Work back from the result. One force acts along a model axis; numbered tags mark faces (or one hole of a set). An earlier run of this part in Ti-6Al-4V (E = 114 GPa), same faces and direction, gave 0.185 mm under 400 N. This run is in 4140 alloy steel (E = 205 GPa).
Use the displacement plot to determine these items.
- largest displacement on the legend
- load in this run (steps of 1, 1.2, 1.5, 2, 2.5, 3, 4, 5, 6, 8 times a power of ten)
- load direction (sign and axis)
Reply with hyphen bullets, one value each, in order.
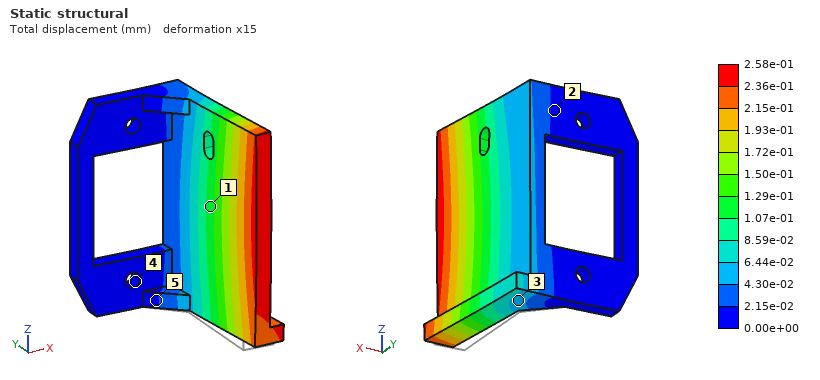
- 2.58e-01 mm
- 1 kN
- +X
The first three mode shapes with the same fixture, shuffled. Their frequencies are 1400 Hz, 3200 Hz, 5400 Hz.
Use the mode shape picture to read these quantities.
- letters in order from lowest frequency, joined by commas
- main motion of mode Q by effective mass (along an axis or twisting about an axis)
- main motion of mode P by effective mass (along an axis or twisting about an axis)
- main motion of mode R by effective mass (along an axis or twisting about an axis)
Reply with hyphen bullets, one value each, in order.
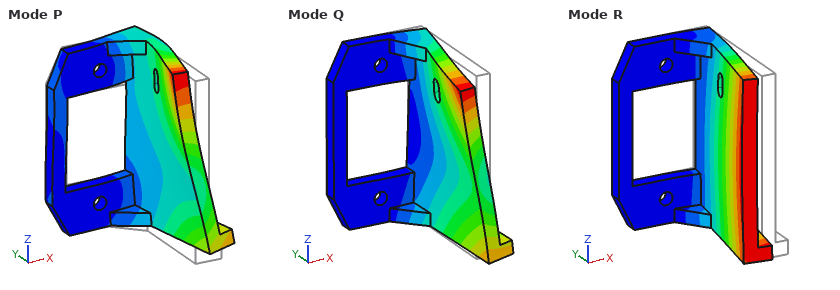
- R, Q, P
- along Z
- along Z
- along X
